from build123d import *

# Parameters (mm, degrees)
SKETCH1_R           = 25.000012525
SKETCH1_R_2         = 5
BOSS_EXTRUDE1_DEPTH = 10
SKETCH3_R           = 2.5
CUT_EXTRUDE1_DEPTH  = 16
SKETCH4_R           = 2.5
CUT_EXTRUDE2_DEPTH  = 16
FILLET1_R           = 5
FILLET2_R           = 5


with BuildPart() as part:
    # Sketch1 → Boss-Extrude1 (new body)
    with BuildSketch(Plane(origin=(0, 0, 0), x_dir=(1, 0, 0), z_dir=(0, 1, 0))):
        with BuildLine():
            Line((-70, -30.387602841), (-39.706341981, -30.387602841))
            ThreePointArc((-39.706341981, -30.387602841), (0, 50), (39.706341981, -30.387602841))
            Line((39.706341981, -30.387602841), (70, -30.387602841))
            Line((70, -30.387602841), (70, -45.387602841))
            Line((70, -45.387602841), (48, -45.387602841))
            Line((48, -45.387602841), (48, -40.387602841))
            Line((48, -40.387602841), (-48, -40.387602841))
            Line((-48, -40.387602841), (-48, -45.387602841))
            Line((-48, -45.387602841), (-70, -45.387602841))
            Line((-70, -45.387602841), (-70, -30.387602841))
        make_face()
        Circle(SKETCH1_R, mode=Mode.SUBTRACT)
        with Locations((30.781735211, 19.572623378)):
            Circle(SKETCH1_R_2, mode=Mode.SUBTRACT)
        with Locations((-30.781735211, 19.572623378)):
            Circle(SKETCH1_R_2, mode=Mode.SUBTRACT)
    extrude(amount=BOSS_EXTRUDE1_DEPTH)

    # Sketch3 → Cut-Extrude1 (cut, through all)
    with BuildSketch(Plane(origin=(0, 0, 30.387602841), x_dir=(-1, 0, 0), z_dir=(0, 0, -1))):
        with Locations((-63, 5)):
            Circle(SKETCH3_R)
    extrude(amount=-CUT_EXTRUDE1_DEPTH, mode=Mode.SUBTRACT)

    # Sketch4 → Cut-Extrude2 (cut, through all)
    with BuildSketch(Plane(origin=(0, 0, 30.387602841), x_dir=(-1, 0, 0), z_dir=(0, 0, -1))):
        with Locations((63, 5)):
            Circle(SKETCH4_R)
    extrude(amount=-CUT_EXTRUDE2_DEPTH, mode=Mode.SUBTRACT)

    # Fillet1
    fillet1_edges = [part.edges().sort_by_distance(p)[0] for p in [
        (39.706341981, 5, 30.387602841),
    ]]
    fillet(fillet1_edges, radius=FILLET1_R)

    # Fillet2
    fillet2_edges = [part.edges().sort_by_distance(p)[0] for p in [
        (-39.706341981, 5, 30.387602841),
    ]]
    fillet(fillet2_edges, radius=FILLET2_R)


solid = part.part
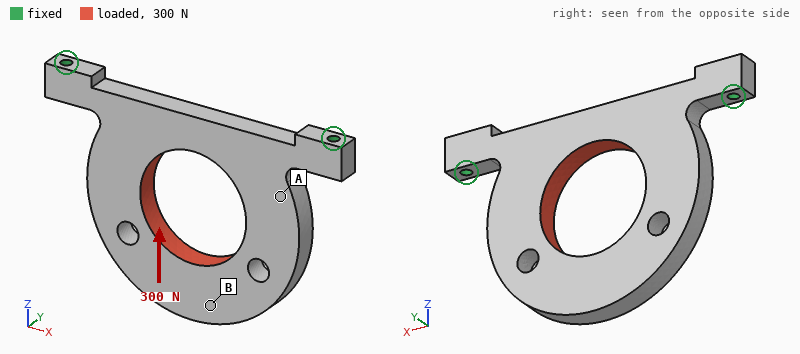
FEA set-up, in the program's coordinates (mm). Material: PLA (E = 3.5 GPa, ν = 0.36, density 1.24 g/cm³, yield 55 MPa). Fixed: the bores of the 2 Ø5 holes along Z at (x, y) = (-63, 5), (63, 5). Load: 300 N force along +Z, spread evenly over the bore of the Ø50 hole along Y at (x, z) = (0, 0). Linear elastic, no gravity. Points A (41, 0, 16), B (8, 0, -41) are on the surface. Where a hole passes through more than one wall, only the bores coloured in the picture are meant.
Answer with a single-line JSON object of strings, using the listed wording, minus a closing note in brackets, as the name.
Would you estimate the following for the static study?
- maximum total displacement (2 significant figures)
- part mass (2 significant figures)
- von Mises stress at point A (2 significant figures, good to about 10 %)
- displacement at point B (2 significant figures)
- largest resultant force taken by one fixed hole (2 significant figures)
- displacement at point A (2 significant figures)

{"maximum total displacement": "68 µm", "part mass": "77 g", "von Mises stress at point A": "1.2 MPa", "displacement at point B": "51 µm", "largest resultant force taken by one fixed hole": "180 N", "displacement at point A": "48 µm"}
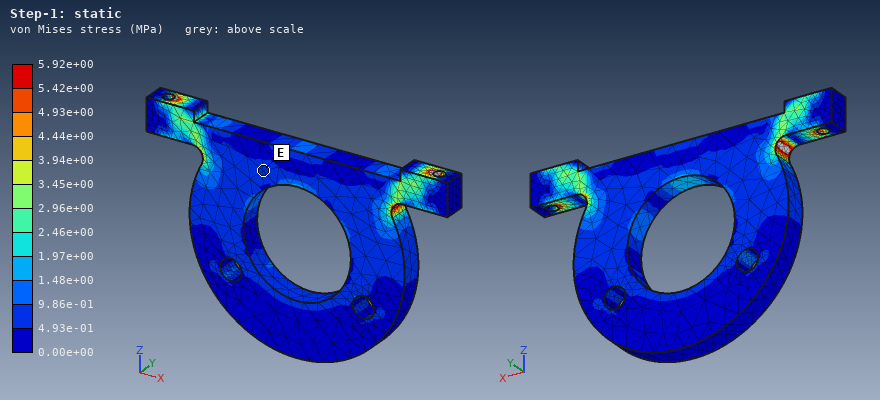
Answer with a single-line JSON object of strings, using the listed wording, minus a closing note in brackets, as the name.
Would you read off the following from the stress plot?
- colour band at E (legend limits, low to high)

{"colour band at E": "4.93e-01 to 9.86e-01 MPa"}
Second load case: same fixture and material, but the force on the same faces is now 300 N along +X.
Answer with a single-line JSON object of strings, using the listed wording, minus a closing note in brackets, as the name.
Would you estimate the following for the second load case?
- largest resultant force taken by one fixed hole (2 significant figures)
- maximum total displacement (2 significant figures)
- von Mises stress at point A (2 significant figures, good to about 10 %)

{"largest resultant force taken by one fixed hole": "180 N", "maximum total displacement": "90 µm", "von Mises stress at point A": "0.97 MPa"}
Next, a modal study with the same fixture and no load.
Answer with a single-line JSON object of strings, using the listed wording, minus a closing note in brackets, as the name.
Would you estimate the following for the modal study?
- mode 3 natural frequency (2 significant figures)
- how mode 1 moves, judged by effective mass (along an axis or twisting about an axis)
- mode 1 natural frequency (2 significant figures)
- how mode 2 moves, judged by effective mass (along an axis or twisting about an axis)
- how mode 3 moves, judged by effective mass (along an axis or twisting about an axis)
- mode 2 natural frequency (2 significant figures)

{"mode 3 natural frequency": "950 Hz", "how mode 1 moves, judged by effective mass": "along Y", "mode 1 natural frequency": "180 Hz", "how mode 2 moves, judged by effective mass": "twisting about Z", "how mode 3 moves, judged by effective mass": "along Y", "mode 2 natural frequency": "680 Hz"}
